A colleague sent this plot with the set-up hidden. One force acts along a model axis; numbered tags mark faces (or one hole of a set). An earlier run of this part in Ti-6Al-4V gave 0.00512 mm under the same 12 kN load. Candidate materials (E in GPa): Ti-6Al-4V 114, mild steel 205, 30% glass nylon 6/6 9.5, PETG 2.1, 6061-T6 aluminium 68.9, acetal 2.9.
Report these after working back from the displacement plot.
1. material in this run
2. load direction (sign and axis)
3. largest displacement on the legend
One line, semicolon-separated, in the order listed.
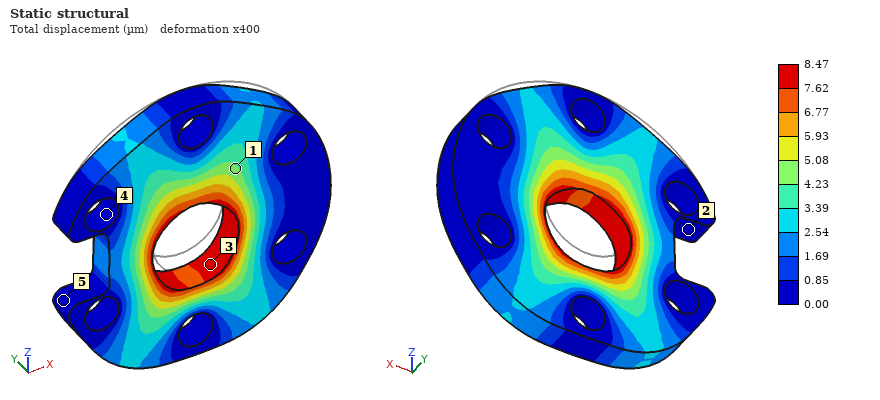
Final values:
6061-T6 aluminium; -Z; 8.47 µm
